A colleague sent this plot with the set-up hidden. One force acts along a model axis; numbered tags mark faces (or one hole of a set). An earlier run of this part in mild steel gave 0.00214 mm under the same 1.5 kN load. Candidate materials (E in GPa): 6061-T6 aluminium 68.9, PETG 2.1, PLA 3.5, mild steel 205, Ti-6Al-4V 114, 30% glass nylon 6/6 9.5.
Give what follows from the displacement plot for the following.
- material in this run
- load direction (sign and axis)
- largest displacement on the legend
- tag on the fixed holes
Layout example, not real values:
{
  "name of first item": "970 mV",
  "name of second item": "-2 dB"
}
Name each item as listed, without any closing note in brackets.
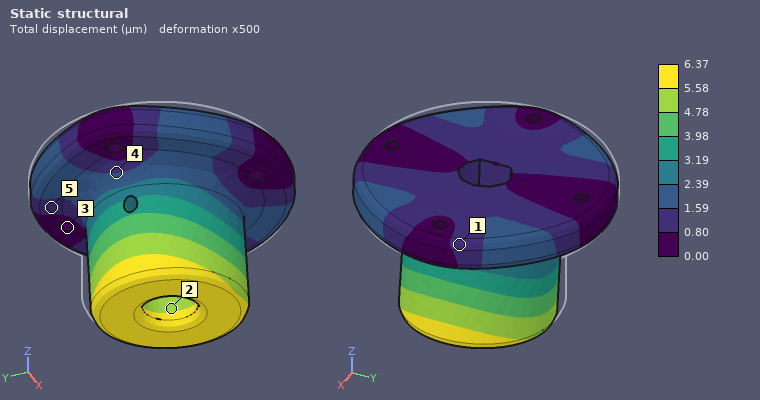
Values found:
{
  "material in this run": "6061-T6 aluminium",
  "load direction": "+X",
  "largest displacement on the legend": "6.37 µm",
  "tag on the fixed holes": "3"
}
